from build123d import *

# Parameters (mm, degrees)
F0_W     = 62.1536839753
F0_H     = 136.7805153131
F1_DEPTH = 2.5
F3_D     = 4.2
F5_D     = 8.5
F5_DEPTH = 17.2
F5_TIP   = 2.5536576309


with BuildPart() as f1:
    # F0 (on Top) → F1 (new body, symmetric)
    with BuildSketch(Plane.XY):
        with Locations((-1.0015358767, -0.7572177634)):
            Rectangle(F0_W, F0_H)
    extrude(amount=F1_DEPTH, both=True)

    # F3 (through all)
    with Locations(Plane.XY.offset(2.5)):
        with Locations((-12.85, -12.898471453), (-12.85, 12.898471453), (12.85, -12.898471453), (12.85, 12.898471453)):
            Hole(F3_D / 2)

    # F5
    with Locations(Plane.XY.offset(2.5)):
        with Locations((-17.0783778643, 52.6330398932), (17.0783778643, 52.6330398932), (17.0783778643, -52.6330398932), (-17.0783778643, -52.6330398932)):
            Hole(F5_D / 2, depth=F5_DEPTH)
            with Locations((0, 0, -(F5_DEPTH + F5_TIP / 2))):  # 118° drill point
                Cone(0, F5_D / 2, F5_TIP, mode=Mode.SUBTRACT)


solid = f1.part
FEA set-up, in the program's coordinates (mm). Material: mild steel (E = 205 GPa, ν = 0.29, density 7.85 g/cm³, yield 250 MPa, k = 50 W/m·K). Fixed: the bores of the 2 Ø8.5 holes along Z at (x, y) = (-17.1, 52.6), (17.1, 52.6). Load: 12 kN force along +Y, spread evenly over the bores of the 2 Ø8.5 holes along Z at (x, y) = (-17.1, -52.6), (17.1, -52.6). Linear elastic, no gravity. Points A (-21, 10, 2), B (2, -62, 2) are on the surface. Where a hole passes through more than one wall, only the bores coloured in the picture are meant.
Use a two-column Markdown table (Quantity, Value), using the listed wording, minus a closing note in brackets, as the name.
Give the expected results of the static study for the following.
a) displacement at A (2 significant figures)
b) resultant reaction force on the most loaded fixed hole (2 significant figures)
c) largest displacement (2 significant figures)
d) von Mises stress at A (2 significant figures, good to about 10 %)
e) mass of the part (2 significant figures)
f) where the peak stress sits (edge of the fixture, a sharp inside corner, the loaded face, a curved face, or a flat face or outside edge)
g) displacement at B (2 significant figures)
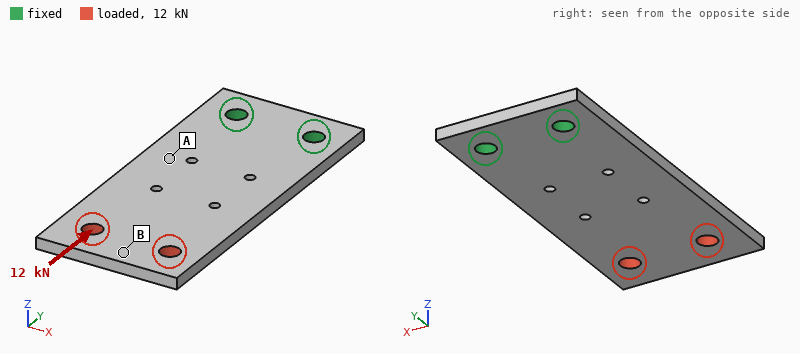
| Quantity | Value |
|---|---|
| displacement at A | 8.5 µm |
| resultant reaction force on the most loaded fixed hole | 6.1 kN |
| largest displacement | 25 µm |
| von Mises stress at A | 39 MPa |
| mass of the part | 320 g |
| where the peak stress sits | a curved face |
| displacement at B | 21 µm |
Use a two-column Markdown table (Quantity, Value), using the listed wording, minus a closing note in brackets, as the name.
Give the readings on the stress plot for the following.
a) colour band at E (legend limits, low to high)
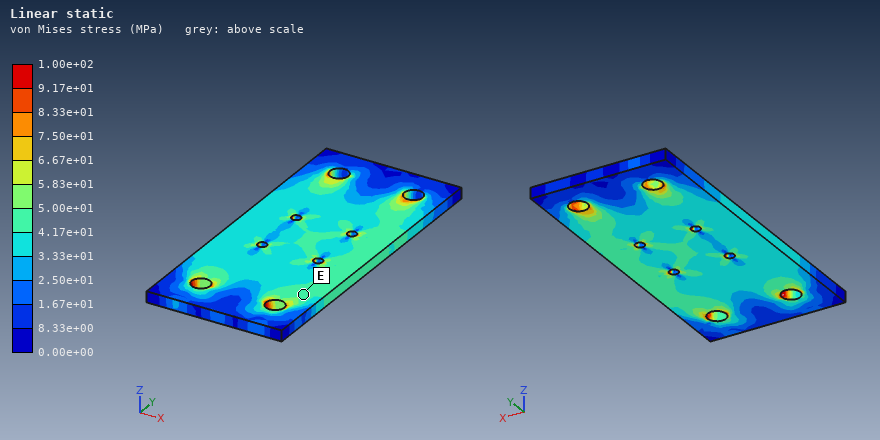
| Quantity | Value |
|---|---|
| colour band at E | 4.17e+01 to 5.00e+01 MPa |
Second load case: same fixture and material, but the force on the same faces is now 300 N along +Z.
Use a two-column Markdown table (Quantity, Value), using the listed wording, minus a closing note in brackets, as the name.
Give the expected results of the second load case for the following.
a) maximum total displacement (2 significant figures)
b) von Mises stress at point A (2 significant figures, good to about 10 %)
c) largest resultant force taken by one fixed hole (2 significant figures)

| Quantity | Value |
|---|---|
| maximum total displacement | 1.0 mm |
| von Mises stress at point A | 76 MPa |
| largest resultant force taken by one fixed hole | 150 N |
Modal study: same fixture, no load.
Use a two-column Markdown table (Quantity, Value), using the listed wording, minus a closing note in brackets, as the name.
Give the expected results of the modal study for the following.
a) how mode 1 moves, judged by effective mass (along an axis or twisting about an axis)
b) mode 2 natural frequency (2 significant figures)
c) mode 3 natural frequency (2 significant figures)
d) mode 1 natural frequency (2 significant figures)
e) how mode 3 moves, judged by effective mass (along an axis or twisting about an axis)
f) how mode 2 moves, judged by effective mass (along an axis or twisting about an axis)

| Quantity | Value |
|---|---|
| how mode 1 moves, judged by effective mass | along Z |
| mode 2 natural frequency | 1200 Hz |
| mode 3 natural frequency | 1800 Hz |
| mode 1 natural frequency | 290 Hz |
| how mode 3 moves, judged by effective mass | along Z |
| how mode 2 moves, judged by effective mass | twisting about Y |
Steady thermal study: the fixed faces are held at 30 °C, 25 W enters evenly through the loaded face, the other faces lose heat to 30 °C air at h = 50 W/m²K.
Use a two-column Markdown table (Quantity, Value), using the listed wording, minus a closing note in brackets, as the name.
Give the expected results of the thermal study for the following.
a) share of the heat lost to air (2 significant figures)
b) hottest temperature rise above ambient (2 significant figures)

| Quantity | Value |
|---|---|
| share of the heat lost to air | 84 % |
| hottest temperature rise above ambient | 63 K |
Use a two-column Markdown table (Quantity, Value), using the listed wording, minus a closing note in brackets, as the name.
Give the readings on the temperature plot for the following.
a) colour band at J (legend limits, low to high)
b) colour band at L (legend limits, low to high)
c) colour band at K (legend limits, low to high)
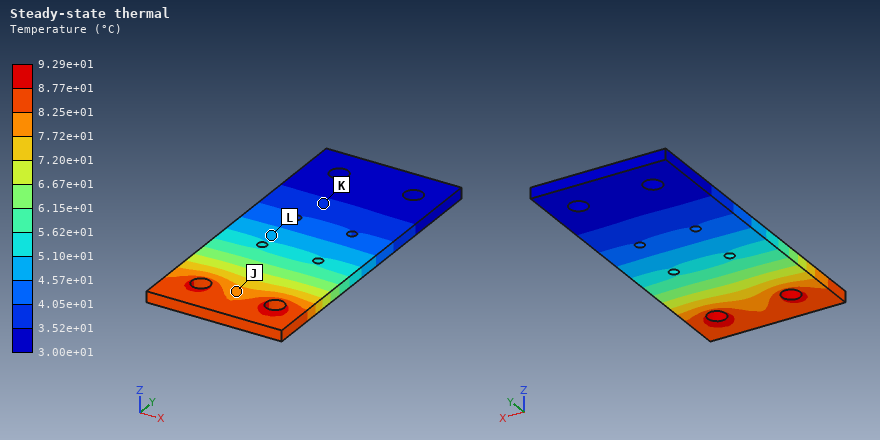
| Quantity | Value |
|---|---|
| colour band at J | 7.72e+01 to 8.25e+01 °C |
| colour band at L | 4.57e+01 to 5.10e+01 °C |
| colour band at K | 3.52e+01 to 4.05e+01 °C |
